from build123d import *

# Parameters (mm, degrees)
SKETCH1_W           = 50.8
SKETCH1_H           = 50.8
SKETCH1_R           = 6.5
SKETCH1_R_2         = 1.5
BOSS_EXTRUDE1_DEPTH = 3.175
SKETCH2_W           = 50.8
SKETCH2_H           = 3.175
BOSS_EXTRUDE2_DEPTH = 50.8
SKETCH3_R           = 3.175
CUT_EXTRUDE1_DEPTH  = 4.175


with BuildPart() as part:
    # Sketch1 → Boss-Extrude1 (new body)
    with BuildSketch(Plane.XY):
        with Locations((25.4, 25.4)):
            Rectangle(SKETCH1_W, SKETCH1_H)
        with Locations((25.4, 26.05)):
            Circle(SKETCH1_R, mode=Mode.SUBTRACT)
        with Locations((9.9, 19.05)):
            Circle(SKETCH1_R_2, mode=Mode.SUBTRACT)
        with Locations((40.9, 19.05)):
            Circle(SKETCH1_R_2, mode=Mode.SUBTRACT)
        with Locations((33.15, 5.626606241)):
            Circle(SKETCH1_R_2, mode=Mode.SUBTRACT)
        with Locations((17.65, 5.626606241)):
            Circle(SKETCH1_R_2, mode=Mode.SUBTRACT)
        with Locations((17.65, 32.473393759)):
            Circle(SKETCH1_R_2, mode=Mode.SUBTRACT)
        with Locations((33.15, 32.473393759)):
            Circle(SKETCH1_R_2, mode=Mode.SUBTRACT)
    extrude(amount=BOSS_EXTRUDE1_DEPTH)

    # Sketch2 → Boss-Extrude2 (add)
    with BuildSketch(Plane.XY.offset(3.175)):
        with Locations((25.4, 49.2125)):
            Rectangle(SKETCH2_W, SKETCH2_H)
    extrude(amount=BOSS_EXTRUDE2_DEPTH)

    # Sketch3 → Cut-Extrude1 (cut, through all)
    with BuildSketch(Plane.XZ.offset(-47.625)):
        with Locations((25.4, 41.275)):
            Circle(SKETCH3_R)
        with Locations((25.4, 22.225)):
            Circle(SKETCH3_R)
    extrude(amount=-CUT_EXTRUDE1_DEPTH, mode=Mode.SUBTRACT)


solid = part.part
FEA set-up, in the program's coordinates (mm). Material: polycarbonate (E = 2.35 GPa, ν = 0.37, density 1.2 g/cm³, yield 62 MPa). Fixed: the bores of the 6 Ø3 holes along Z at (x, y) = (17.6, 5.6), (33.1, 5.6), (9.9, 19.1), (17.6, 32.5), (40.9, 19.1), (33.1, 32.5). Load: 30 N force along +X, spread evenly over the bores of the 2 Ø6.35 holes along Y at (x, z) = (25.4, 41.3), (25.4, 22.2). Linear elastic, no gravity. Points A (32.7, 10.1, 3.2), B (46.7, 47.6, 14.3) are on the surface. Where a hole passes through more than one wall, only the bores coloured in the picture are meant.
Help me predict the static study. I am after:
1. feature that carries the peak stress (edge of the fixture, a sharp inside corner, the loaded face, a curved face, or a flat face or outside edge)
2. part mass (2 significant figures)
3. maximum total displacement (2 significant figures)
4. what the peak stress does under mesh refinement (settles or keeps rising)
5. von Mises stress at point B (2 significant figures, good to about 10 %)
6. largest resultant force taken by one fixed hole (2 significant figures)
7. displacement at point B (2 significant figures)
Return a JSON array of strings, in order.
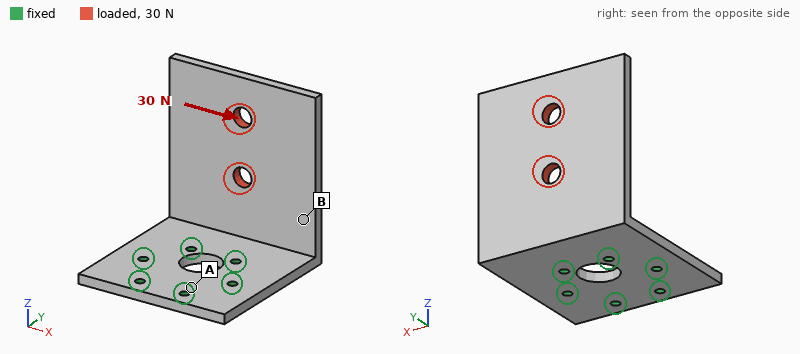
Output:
["edge of the fixture", "19 g", "0.91 mm", "keeps rising", "2.3 MPa", "43 N", "0.38 mm"]
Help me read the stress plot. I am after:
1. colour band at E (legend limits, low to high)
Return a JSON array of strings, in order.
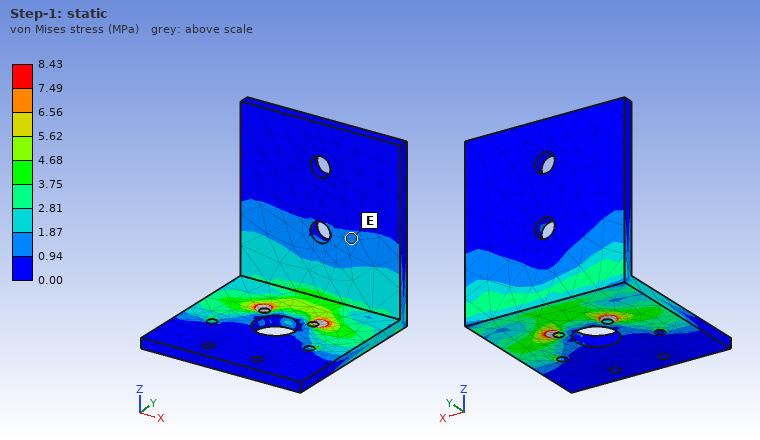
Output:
["0.94 to 1.87 MPa"]
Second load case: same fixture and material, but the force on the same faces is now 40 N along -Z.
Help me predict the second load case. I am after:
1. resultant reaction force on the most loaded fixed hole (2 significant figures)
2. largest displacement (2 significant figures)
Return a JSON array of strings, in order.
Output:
["28 N", "1.0 mm"]
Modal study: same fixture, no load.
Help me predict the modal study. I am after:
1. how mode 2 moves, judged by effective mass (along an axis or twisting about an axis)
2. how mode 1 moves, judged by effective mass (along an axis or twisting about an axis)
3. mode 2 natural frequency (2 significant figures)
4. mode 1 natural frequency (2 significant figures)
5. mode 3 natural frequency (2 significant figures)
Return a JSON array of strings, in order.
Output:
["along X", "along Y", "350 Hz", "180 Hz", "610 Hz"]
